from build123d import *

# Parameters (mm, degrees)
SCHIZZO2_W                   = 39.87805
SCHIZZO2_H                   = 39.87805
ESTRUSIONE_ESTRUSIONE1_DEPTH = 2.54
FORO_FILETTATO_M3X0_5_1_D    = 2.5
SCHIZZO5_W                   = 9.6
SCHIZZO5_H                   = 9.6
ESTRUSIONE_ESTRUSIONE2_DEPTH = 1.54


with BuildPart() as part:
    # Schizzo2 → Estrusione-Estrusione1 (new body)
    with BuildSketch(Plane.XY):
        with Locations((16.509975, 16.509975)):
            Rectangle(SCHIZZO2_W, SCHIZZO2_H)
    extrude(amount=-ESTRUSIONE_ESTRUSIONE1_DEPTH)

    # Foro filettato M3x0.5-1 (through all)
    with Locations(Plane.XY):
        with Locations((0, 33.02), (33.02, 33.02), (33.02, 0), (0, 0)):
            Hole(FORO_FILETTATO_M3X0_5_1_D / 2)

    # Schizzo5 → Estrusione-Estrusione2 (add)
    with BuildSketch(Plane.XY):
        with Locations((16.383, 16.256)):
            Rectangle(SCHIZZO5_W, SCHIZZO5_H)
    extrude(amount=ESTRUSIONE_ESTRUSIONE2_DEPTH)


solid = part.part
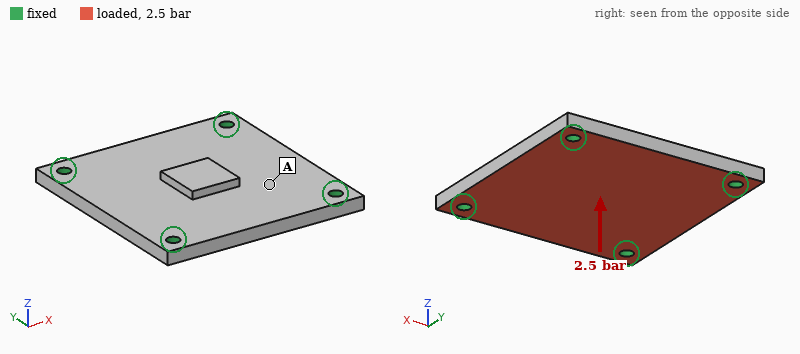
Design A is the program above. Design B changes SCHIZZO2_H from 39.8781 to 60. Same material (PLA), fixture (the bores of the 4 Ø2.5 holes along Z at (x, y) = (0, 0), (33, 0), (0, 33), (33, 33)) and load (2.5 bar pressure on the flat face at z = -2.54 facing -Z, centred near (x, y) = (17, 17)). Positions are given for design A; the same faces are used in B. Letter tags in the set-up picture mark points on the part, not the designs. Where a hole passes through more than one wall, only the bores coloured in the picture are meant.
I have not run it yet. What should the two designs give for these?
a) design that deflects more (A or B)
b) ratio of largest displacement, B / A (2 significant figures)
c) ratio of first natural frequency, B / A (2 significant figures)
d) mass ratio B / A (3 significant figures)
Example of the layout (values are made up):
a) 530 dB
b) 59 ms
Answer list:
a) B
b) 1.3
c) 0.95
d) 1.49
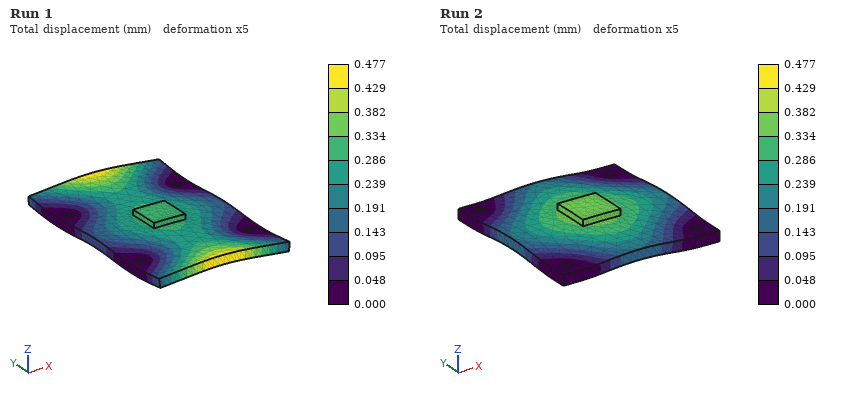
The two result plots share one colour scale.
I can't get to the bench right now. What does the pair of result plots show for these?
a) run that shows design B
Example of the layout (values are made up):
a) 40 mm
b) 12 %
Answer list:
a) Run 1
